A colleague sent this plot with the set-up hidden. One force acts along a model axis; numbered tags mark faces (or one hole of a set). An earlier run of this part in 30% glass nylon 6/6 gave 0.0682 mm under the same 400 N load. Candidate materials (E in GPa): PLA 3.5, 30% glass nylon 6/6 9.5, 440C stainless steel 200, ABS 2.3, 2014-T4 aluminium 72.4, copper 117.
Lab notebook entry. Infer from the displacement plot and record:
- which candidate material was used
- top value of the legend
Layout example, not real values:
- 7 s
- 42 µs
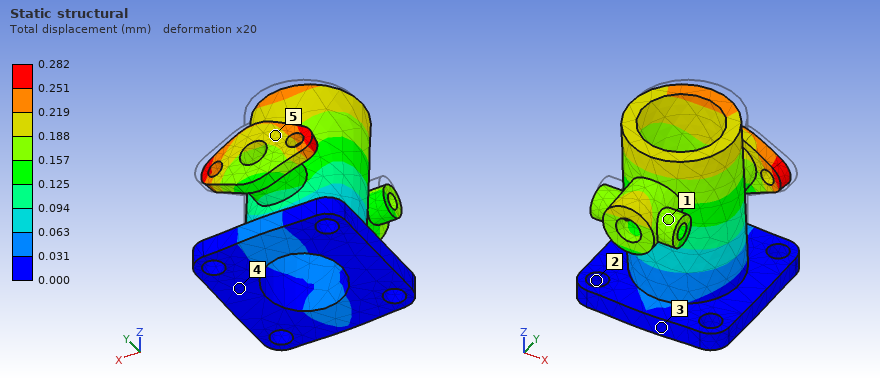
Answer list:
- ABS
- 0.282 mm
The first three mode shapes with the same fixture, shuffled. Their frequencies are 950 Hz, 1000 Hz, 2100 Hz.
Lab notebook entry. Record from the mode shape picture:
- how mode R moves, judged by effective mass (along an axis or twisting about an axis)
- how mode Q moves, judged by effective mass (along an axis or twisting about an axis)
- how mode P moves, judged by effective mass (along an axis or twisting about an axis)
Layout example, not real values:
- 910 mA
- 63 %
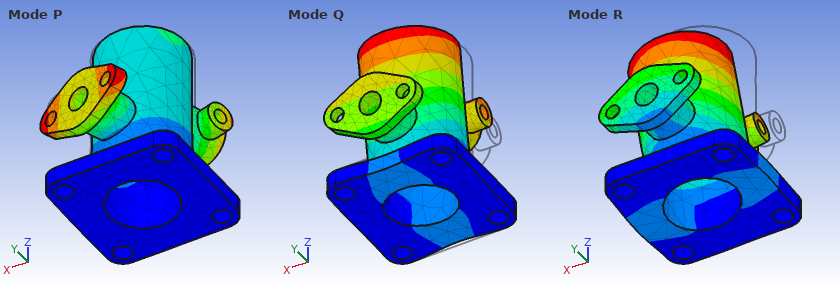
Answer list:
- along X
- along Y
- twisting about Z
